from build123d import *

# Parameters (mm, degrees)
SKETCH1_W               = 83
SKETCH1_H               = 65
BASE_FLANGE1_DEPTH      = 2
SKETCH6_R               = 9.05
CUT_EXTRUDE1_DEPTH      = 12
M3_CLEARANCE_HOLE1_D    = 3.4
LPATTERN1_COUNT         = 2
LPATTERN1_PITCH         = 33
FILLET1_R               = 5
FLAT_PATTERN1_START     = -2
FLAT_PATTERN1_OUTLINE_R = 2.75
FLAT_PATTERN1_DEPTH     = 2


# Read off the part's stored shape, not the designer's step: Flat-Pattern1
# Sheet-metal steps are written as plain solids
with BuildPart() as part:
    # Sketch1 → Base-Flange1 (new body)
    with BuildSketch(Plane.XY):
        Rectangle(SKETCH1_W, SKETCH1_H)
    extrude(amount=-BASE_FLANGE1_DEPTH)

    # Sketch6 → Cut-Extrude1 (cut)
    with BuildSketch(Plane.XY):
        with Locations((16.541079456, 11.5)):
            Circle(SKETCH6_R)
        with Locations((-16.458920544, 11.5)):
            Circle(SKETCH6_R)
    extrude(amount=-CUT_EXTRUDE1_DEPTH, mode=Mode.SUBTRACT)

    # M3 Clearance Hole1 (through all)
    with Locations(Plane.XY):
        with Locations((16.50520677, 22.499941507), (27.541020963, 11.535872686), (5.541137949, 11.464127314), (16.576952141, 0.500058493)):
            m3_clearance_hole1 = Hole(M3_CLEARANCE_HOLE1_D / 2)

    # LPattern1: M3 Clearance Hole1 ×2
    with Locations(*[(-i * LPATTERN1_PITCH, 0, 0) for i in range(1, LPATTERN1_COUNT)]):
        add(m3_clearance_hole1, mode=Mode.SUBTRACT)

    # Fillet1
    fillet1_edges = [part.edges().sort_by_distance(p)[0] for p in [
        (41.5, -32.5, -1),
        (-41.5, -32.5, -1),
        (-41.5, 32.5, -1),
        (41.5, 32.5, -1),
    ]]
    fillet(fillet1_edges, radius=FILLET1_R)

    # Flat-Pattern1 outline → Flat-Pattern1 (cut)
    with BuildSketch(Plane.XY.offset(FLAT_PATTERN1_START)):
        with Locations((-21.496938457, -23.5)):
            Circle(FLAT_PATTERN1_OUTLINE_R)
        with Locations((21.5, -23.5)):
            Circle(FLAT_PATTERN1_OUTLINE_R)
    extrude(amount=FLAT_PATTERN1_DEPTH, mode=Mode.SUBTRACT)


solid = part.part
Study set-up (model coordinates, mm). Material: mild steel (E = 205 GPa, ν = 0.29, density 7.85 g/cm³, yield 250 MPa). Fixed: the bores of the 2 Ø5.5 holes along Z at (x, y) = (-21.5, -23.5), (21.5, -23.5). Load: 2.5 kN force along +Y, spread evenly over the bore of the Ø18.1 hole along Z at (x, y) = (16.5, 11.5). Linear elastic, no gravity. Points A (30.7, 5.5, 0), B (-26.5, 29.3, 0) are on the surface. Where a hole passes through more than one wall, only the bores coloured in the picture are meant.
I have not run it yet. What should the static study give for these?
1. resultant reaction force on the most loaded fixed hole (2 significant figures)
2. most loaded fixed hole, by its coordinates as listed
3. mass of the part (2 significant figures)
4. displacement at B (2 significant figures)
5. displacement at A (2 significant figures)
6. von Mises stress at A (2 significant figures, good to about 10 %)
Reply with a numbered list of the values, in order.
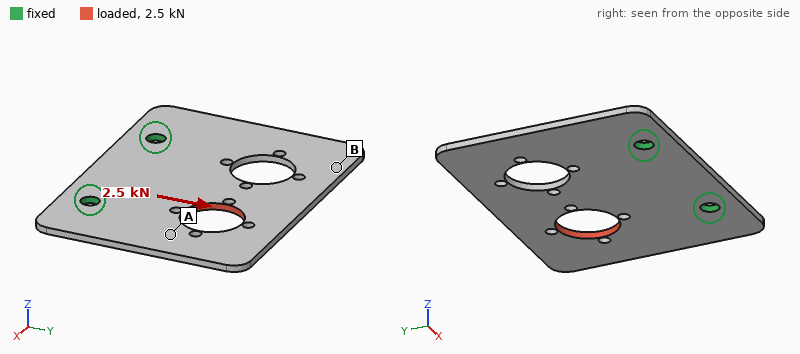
1. 2.1 kN
2. (21.5, -23.5)
3. 74 g
4. 6.1 µm
5. 9.2 µm
6. 31 MPa
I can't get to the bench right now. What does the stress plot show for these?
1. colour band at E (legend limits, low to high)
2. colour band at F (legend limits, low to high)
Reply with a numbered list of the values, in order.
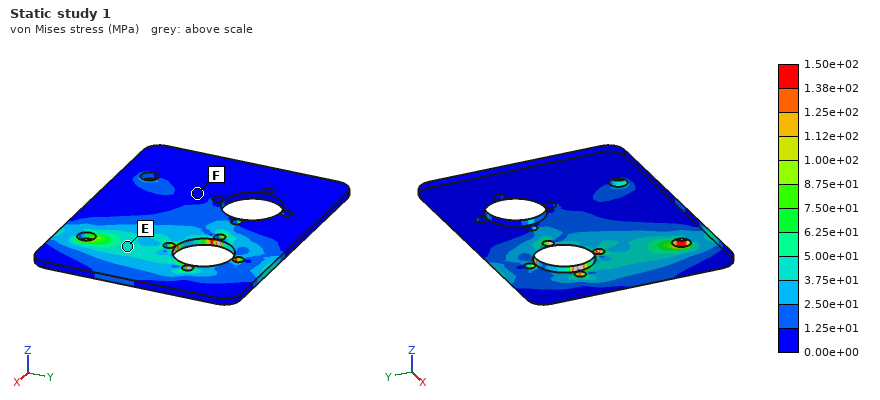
1. 3.75e+01 to 5.00e+01 MPa
2. 0.00e+00 to 1.25e+01 MPa
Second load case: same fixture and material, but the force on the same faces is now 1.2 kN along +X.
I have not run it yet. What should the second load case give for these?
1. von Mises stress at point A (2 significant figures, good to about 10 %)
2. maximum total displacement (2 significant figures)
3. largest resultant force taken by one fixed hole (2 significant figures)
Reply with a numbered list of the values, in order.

1. 16 MPa
2. 15 µm
3. 1.1 kN
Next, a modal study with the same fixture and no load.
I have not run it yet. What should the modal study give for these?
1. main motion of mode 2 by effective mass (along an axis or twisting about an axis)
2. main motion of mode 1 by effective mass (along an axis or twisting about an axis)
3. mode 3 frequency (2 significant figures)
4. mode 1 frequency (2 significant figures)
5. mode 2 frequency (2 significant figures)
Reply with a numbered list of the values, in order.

1. twisting about Y
2. along Z
3. 1900 Hz
4. 540 Hz
5. 900 Hz
